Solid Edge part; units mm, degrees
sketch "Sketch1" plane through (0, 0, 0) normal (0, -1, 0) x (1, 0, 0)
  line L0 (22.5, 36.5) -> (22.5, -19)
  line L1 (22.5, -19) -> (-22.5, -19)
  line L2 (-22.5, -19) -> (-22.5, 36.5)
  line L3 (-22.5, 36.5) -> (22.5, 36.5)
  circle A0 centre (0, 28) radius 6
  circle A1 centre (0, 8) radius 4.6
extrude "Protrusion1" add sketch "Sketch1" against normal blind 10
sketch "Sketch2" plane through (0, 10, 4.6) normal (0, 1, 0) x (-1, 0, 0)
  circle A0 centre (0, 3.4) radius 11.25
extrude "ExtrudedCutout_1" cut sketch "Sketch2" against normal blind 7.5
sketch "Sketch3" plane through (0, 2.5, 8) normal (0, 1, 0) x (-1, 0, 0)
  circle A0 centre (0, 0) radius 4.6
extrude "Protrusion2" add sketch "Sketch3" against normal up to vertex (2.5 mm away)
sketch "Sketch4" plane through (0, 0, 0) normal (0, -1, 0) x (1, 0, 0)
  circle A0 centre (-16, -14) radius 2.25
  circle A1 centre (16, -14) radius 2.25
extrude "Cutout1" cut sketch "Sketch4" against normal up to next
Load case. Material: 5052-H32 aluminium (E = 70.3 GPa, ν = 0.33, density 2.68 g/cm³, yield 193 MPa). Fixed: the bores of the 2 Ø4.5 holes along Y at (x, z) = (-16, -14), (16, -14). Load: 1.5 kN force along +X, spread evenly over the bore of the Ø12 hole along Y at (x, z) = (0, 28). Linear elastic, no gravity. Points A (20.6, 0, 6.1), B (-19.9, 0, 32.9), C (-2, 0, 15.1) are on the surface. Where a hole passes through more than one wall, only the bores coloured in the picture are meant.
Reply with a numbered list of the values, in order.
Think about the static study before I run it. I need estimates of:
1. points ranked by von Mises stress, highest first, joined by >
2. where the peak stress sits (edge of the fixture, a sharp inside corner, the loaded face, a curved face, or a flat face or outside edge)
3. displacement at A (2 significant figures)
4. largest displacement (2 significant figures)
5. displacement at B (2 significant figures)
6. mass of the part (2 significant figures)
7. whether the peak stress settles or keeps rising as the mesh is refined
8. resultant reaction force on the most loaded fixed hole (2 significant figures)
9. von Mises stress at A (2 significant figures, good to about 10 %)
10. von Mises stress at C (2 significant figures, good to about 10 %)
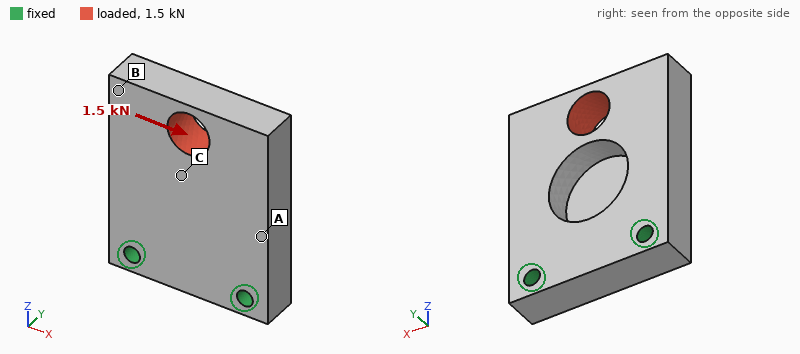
1. C > A > B
2. edge of the fixture
3. 11 µm
4. 34 µm
5. 27 µm
6. 55 g
7. keeps rising
8. 1.9 kN
9. 14 MPa
10. 26 MPa
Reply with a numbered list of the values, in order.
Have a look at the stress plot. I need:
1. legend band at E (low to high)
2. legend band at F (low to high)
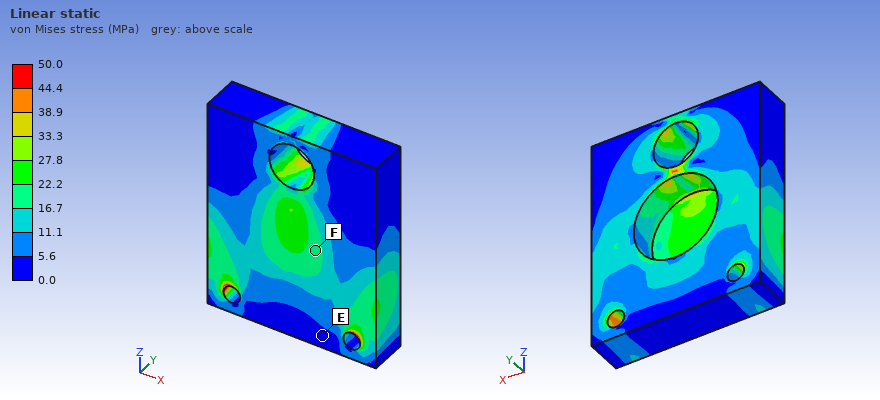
1. 0.0 to 5.6 MPa
2. 16.7 to 22.2 MPa
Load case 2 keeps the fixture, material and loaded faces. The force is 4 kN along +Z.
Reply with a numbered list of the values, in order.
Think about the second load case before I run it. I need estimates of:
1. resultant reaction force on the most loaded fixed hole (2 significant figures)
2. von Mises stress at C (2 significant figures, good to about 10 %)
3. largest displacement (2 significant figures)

1. 2.0 kN
2. 22 MPa
3. 27 µm
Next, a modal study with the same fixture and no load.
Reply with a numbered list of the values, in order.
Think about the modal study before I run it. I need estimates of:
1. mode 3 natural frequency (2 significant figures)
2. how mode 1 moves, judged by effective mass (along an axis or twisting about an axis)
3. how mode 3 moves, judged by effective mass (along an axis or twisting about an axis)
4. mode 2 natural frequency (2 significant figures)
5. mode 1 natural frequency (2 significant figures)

1. 8800 Hz
2. along Y
3. along X
4. 6200 Hz
5. 2900 Hz
